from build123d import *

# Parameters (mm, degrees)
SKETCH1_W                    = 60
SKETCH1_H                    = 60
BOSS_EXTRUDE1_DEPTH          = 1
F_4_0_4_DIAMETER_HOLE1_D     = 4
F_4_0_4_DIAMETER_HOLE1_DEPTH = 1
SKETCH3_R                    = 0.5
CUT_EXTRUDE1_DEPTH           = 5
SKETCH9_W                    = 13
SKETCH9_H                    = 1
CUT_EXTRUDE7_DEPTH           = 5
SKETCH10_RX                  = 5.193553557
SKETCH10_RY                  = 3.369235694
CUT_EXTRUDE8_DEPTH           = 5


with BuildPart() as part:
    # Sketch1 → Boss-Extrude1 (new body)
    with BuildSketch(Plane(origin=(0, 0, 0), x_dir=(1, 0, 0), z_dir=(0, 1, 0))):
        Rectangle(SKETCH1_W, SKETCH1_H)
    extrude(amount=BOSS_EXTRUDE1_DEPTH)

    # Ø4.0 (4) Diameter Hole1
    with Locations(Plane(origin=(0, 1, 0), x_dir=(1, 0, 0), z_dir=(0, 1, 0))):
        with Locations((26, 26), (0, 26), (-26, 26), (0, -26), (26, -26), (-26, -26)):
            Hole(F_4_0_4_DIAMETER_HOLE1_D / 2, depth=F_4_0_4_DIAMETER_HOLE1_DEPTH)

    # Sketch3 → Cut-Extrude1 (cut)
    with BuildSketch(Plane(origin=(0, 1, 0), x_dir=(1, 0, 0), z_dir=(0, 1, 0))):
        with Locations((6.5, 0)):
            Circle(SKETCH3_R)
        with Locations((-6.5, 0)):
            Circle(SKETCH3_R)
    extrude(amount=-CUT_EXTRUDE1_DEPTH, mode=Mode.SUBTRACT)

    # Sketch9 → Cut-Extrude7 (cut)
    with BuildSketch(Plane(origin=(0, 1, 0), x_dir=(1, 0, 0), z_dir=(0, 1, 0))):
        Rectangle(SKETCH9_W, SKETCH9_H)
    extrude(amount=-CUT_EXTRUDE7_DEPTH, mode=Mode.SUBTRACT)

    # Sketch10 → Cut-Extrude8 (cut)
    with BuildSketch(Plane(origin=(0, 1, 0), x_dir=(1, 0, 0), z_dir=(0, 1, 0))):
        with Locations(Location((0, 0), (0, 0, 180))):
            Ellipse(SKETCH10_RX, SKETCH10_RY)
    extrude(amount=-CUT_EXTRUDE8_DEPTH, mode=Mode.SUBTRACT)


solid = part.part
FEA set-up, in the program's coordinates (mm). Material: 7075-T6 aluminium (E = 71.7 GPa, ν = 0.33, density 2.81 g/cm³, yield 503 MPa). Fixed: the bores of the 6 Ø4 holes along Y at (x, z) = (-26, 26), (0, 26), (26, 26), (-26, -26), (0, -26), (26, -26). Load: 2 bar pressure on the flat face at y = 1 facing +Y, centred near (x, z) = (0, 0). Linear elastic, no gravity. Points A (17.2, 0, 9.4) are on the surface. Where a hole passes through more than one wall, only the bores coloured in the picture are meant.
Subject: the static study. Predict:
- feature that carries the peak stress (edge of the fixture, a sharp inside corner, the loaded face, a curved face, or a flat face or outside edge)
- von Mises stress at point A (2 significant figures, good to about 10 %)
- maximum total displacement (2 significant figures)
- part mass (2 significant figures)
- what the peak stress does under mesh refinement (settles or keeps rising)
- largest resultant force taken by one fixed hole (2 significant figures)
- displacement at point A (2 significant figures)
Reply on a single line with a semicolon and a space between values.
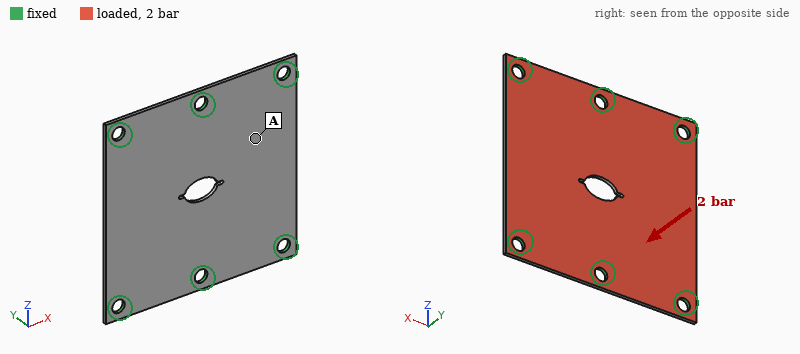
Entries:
edge of the fixture; 69 MPa; 0.70 mm; 9.7 g; keeps rising; 150 N; 0.48 mm
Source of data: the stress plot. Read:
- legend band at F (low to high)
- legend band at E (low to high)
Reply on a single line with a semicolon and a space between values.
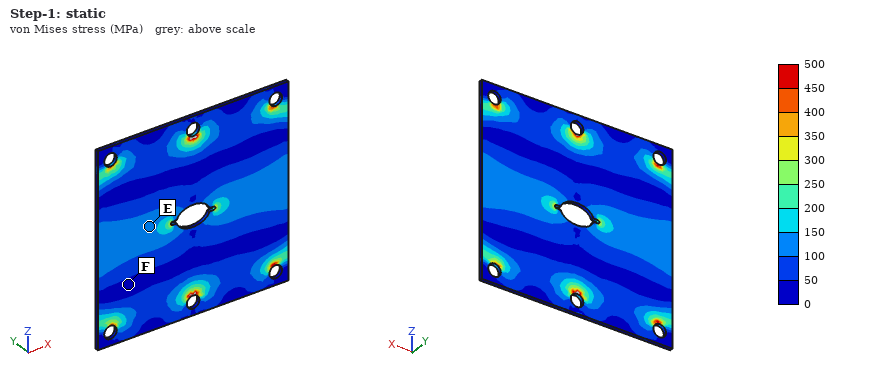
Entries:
0 to 50 MPa; 100 to 150 MPa
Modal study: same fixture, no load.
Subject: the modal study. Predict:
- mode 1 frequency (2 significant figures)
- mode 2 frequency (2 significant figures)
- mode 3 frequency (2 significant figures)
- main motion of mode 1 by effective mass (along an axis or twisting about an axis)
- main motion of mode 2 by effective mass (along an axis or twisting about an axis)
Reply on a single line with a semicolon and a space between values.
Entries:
1900 Hz; 2300 Hz; 3500 Hz; along Y; twisting about Z
